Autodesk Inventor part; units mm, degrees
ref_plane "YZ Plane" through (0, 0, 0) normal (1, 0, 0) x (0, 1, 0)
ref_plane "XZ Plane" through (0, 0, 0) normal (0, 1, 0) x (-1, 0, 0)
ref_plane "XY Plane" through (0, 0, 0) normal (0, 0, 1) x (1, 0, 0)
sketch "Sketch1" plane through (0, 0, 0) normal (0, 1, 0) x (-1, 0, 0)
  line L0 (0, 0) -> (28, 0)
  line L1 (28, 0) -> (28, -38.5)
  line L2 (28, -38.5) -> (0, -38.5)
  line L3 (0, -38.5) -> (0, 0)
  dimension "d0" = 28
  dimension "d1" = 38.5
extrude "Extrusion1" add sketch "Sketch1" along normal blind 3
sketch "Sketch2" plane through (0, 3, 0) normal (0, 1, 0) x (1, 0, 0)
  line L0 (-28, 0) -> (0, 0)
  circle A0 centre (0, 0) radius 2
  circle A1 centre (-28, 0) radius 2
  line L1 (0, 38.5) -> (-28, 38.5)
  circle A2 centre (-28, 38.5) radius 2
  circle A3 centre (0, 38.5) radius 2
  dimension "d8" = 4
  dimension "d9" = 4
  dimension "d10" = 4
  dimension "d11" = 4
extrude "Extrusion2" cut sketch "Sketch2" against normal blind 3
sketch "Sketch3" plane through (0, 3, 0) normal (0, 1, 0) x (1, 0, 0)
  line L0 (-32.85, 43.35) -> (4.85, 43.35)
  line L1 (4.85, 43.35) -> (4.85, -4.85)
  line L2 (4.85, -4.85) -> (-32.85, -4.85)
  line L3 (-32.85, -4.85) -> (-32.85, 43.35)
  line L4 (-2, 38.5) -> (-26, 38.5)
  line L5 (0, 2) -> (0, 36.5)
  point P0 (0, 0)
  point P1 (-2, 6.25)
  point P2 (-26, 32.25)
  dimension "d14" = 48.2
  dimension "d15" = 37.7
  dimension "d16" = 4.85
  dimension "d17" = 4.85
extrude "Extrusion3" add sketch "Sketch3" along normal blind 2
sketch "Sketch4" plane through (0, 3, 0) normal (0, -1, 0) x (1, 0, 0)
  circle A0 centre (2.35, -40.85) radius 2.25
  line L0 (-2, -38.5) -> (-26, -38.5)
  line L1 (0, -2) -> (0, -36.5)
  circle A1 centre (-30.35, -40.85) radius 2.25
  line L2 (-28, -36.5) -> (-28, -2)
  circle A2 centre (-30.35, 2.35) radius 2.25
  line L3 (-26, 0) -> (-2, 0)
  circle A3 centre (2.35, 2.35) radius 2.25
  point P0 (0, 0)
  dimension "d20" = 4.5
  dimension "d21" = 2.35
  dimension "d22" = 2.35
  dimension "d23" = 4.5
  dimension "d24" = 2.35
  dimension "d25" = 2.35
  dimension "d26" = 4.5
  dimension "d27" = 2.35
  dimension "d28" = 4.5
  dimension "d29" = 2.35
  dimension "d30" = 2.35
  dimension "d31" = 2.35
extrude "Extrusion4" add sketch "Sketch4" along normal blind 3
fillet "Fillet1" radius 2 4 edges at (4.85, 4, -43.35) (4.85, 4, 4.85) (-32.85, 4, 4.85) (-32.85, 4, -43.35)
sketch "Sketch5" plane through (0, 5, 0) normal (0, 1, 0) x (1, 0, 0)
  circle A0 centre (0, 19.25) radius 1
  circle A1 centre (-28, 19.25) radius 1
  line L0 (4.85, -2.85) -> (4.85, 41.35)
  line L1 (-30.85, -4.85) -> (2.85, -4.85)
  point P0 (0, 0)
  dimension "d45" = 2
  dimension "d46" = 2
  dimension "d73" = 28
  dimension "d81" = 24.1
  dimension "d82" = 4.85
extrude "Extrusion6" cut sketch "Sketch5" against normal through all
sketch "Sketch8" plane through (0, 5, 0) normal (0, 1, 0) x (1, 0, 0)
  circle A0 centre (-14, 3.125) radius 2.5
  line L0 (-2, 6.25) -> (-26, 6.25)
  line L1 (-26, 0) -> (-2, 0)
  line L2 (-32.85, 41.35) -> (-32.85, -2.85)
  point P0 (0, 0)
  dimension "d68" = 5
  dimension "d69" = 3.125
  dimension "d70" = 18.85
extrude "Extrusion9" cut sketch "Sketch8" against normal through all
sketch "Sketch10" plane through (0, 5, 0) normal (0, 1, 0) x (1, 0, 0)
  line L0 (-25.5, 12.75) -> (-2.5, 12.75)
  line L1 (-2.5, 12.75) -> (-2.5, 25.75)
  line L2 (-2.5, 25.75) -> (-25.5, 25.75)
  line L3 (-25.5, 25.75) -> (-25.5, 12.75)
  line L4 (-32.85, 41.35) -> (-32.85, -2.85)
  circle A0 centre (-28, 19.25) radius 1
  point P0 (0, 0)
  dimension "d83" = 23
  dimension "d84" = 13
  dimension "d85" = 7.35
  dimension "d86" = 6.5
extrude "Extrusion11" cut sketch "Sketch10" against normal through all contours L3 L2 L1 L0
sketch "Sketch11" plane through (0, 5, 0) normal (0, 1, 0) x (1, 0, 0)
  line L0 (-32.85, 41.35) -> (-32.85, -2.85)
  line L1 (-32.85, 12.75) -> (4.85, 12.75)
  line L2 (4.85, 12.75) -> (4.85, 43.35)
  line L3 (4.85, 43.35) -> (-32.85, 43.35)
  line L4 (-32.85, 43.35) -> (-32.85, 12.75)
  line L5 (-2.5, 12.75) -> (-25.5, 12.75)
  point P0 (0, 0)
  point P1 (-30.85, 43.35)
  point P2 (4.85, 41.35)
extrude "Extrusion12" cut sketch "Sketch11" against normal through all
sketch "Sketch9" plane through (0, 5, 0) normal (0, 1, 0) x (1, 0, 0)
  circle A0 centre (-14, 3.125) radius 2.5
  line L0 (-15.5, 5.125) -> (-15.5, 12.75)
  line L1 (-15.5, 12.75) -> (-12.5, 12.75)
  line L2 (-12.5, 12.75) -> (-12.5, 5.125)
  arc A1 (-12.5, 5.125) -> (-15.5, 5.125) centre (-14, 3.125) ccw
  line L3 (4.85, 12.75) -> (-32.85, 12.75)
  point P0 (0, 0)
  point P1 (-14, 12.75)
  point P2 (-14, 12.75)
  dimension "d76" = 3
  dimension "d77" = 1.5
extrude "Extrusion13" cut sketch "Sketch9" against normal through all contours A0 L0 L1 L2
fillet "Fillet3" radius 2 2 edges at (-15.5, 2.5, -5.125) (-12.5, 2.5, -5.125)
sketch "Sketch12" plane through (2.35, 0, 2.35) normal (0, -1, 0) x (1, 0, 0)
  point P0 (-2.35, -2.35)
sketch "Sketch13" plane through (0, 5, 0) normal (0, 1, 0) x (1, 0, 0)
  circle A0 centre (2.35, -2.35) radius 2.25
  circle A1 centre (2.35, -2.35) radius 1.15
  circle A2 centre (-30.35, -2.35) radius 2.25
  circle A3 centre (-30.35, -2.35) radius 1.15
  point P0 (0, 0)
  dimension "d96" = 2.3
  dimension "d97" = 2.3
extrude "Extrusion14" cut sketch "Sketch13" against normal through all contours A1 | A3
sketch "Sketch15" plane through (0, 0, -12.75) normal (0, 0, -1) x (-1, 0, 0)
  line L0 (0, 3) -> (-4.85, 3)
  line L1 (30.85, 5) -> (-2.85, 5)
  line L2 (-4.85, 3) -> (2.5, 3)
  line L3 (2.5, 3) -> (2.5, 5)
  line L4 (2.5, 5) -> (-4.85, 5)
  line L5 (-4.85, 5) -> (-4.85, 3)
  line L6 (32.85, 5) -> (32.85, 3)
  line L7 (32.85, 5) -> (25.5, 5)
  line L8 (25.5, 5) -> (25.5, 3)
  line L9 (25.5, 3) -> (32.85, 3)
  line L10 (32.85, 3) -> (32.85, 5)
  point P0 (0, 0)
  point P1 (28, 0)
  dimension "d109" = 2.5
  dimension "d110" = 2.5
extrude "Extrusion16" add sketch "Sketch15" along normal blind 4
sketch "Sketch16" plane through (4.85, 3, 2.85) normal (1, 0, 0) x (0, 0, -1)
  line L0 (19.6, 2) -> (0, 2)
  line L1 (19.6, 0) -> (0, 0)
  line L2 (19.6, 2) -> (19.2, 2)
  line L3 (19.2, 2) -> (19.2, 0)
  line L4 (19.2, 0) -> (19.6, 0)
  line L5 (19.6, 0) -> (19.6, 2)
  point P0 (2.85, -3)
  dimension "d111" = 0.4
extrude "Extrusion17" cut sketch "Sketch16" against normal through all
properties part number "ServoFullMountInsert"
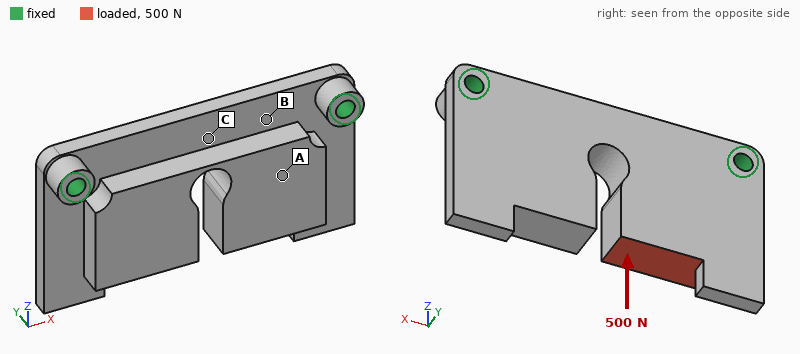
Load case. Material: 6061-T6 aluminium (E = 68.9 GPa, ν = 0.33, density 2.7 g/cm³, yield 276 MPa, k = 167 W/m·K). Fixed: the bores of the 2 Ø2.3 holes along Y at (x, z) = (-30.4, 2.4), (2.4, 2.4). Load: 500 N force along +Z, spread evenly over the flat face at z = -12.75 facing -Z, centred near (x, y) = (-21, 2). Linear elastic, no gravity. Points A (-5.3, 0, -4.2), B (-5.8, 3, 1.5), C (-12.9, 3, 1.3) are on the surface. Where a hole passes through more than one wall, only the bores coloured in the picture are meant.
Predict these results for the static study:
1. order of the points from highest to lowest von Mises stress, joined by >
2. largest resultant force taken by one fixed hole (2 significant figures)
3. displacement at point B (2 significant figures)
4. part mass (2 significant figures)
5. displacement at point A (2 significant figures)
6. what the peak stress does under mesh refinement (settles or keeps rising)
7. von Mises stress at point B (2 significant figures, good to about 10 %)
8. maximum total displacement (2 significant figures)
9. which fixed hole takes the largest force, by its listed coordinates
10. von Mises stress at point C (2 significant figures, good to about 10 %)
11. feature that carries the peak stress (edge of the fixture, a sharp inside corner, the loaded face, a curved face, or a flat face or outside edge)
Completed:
C > B > A
380 N
0.015 mm
6.3 g
0.024 mm
keeps rising
32 MPa
0.10 mm
(-30.4, 2.4)
65 MPa
a sharp inside corner
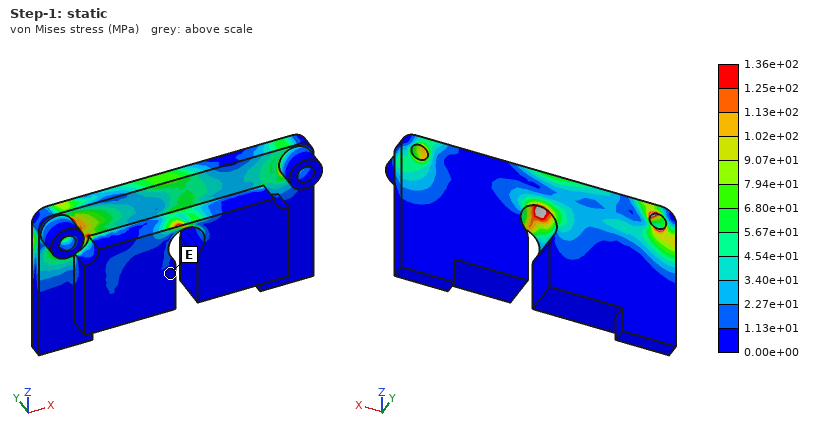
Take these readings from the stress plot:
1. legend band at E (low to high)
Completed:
0.00e+00 to 1.13e+01 MPa
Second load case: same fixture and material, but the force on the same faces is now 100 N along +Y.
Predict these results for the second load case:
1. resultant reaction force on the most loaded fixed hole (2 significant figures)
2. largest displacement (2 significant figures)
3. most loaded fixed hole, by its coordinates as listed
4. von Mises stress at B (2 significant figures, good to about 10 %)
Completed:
84 N
0.16 mm
(-30.4, 2.4)
20 MPa
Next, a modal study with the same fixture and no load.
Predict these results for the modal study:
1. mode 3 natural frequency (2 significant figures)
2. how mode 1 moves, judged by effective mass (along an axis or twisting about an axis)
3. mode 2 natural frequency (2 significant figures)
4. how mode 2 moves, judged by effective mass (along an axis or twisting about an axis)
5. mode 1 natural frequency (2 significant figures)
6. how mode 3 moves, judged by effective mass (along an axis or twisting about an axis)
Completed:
8500 Hz
along Y
5300 Hz
twisting about Z
3700 Hz
along Z
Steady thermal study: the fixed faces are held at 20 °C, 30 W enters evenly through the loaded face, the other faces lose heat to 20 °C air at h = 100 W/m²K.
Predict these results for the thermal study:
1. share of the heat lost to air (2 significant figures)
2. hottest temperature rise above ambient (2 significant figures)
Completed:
15 %
68 K
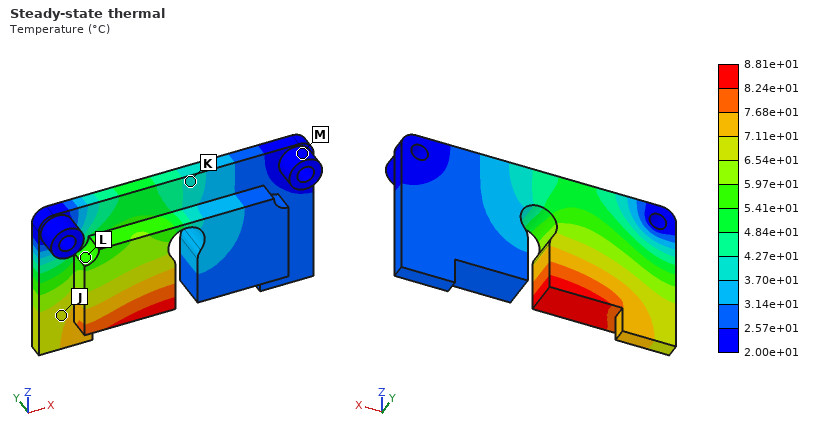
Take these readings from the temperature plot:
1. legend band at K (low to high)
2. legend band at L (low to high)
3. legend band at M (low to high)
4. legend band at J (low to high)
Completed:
3.70e+01 to 4.27e+01 °C
5.41e+01 to 5.97e+01 °C
2.00e+01 to 2.57e+01 °C
6.54e+01 to 7.11e+01 °C
